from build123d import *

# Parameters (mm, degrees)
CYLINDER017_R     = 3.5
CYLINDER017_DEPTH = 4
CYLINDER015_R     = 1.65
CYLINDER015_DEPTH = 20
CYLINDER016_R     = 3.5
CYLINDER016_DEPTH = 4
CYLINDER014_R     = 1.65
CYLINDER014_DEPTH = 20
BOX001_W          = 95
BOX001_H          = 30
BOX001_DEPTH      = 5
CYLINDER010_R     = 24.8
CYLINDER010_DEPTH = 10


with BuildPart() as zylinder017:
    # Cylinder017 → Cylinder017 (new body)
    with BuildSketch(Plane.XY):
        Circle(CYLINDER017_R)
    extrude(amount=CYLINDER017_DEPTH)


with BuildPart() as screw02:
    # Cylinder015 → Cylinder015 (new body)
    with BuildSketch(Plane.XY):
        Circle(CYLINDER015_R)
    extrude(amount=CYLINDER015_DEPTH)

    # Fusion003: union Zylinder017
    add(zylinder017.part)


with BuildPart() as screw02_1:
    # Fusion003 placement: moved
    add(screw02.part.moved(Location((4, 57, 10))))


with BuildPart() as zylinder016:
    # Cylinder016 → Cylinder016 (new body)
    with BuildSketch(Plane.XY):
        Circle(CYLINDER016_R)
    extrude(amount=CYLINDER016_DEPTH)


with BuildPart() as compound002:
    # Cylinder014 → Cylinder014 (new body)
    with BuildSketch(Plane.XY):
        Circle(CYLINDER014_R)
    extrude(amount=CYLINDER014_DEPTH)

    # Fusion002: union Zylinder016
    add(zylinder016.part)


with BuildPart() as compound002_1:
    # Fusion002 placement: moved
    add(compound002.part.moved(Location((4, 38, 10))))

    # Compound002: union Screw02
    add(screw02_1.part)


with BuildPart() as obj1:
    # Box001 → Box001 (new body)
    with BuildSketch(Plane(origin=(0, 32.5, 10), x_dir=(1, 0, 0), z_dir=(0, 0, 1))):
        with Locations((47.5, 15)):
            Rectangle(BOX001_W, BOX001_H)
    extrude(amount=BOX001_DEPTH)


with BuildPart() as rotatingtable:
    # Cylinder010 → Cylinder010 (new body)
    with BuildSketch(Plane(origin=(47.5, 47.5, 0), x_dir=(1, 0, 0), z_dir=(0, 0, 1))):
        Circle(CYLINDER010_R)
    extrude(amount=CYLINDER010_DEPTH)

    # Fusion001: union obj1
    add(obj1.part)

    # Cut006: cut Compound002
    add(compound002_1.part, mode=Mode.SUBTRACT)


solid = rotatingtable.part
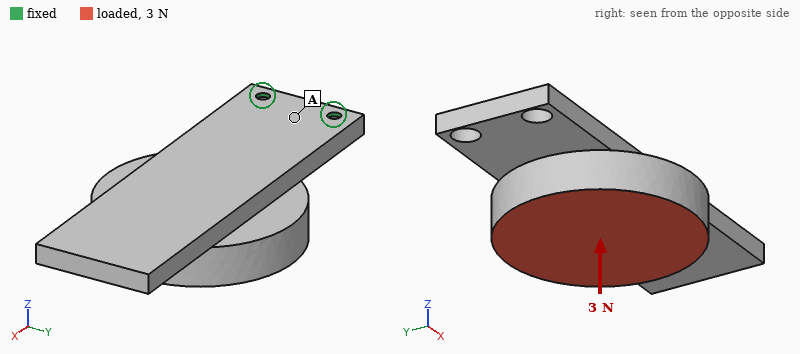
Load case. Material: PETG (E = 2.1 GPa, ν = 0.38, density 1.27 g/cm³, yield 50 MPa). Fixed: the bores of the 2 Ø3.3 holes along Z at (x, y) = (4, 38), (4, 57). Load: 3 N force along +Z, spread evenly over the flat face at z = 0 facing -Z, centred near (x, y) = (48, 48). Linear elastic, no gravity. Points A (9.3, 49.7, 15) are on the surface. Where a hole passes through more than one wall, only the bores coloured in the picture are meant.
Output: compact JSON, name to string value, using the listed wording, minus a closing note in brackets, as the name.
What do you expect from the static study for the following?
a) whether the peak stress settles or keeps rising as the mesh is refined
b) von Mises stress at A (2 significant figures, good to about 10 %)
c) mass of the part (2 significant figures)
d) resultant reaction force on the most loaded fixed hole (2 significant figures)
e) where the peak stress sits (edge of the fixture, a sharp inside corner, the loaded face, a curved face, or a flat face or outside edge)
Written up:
{"whether the peak stress settles or keeps rising as the mesh is refined": "keeps rising", "von Mises stress at A": "0.95 MPa", "mass of the part": "42 g", "resultant reaction force on the most loaded fixed hole": "2.0 N", "where the peak stress sits": "edge of the fixture"}
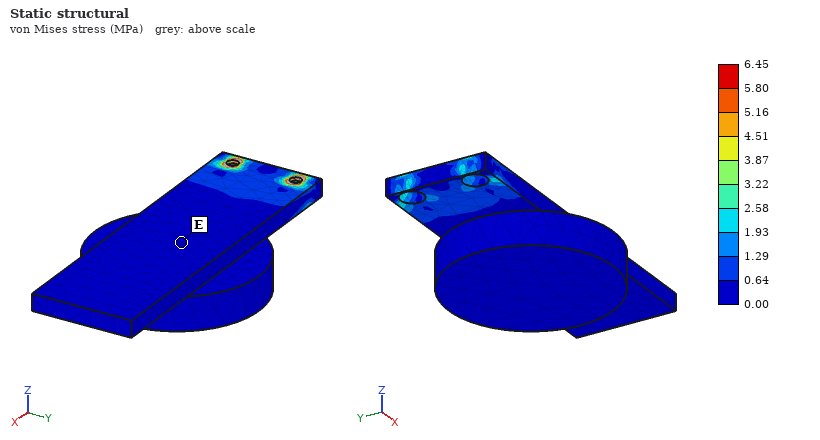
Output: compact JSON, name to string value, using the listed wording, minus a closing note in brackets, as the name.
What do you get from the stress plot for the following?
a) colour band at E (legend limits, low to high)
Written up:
{"colour band at E": "0.00 to 0.64 MPa"}
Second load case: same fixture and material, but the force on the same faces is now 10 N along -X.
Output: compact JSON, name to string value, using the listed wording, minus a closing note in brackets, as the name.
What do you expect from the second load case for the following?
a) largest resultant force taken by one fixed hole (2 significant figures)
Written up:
{"largest resultant force taken by one fixed hole": "5.1 N"}
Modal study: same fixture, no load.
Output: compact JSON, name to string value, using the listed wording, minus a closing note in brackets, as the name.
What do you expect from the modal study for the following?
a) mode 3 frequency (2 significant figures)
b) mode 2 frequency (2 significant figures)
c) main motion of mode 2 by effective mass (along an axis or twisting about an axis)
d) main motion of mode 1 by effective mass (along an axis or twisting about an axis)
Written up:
{"mode 3 frequency": "440 Hz", "mode 2 frequency": "360 Hz", "main motion of mode 2 by effective mass": "along Y", "main motion of mode 1 by effective mass": "along Z"}
